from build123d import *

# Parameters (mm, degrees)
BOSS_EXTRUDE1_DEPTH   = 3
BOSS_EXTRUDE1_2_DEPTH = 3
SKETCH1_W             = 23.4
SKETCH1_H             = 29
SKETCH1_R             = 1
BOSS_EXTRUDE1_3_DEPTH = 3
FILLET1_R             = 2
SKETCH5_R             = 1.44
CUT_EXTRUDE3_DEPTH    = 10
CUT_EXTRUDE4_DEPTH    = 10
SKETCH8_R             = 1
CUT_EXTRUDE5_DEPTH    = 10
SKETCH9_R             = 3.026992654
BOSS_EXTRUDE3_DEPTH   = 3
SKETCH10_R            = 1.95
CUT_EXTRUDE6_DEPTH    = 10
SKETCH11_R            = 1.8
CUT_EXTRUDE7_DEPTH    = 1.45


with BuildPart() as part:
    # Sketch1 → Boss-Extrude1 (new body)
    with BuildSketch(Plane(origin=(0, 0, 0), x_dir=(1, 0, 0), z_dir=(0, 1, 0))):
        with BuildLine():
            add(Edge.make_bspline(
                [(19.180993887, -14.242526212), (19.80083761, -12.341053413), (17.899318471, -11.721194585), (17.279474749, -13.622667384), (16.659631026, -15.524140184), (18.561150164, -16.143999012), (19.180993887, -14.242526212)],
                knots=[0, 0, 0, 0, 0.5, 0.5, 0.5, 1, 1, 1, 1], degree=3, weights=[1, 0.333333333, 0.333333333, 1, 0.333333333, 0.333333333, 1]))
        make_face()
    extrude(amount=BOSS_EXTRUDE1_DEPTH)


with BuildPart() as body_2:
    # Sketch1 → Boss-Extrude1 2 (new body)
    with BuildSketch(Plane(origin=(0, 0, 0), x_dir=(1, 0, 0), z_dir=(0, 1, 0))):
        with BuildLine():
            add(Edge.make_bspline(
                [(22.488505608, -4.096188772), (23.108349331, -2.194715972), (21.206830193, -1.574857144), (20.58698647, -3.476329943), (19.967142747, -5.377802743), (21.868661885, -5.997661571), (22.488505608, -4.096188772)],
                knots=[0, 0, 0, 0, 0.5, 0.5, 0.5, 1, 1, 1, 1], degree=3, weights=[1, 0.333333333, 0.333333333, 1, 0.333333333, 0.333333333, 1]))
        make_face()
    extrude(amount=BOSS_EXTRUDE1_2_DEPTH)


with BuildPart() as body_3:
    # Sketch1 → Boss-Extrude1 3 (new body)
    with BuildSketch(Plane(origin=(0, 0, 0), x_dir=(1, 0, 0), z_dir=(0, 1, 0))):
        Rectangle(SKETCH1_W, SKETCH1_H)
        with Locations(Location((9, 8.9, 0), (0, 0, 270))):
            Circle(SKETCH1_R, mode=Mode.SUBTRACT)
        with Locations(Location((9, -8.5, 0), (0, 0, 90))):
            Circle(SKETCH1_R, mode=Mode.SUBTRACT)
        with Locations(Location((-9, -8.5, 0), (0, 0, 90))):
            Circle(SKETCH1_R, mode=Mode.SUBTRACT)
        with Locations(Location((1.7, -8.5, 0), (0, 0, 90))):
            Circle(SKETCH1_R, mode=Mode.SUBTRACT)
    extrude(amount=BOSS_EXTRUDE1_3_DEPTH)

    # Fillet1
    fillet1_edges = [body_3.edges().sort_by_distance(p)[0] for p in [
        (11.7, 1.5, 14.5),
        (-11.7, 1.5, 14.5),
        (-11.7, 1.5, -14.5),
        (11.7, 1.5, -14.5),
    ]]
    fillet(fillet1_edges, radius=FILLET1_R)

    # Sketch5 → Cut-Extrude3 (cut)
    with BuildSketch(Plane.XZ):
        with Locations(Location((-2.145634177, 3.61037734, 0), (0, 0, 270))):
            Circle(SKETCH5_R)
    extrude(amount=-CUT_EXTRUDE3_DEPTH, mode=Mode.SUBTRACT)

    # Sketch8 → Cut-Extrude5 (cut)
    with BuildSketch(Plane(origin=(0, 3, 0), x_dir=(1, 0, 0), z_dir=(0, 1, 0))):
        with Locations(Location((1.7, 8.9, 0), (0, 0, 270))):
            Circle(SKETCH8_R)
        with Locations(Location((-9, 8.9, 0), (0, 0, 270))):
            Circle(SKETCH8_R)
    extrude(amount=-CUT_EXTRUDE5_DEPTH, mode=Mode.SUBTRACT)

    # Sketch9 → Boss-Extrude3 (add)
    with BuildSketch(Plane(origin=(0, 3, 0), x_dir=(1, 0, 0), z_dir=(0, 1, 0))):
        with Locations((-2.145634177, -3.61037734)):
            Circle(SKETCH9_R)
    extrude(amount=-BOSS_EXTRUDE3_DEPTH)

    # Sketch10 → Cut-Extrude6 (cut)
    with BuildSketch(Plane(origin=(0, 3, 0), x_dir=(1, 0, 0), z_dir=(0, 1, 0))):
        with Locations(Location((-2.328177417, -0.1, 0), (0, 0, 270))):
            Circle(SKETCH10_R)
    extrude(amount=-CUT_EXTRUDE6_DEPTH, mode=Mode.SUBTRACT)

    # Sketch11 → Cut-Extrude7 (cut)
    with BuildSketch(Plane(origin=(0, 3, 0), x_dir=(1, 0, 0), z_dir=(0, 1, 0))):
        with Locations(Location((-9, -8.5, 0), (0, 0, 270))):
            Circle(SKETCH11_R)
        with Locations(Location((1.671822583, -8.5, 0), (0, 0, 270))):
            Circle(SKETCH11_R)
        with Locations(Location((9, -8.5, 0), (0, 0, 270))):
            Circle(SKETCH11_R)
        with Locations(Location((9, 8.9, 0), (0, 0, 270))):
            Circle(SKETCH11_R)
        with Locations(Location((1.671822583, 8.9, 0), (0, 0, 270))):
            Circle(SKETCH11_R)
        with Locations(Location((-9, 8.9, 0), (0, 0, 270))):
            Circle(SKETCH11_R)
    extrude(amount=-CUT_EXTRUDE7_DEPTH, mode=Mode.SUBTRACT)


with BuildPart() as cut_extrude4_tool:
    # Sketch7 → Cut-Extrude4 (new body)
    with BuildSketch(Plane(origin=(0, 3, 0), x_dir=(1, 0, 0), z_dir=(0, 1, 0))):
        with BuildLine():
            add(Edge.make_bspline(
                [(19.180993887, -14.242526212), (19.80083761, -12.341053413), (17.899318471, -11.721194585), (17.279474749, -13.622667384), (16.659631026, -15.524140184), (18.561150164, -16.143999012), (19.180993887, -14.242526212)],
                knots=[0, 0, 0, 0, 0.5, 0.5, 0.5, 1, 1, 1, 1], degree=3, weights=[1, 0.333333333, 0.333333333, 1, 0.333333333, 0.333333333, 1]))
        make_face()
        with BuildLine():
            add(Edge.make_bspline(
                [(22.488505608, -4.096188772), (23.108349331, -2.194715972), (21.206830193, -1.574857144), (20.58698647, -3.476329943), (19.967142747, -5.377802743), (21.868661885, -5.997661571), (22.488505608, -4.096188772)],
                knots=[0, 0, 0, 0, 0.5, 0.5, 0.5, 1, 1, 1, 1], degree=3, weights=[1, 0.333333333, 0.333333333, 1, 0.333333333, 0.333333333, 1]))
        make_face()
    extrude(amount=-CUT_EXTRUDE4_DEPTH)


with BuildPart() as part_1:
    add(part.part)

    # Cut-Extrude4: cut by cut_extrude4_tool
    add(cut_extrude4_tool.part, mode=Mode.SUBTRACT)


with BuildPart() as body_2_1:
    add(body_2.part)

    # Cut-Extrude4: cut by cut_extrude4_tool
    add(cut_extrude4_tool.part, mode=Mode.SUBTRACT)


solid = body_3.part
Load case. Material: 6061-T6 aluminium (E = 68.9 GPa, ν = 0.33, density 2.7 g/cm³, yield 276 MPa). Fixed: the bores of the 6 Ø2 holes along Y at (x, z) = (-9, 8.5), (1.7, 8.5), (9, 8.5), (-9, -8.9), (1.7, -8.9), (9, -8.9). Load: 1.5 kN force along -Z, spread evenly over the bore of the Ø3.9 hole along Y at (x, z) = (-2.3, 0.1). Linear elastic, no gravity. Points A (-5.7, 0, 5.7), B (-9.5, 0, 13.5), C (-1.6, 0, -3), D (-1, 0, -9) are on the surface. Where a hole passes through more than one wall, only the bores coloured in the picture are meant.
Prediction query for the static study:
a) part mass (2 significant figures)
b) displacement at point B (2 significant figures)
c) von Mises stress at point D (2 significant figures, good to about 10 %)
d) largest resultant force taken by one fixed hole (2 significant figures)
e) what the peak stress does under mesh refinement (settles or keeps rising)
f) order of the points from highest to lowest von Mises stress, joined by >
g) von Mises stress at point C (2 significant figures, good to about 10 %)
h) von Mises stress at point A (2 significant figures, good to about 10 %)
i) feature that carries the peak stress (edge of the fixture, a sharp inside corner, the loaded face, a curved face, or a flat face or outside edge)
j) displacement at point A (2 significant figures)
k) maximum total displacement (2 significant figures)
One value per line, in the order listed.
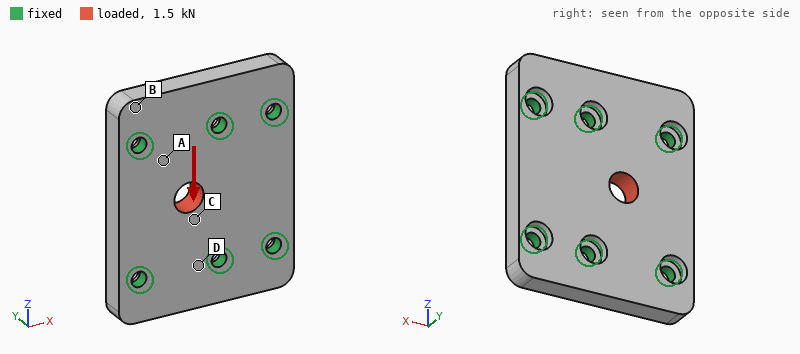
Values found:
5.1 g
1.7 µm
14 MPa
370 N
keeps rising
C > A > D > B
38 MPa
26 MPa
edge of the fixture
1.8 µm
4.4 µm
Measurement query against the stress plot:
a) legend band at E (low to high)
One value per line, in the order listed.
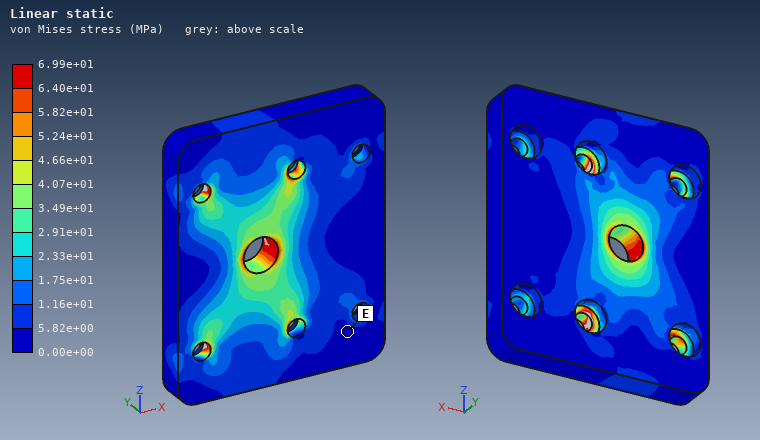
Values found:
0.00e+00 to 5.82e+00 MPa
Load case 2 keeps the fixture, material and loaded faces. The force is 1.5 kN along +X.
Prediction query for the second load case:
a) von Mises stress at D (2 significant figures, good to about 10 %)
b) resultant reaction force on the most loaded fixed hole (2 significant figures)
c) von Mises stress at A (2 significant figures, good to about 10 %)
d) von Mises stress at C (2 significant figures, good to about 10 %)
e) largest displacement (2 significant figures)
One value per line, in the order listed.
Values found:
16 MPa
330 N
30 MPa
34 MPa
6.0 µm
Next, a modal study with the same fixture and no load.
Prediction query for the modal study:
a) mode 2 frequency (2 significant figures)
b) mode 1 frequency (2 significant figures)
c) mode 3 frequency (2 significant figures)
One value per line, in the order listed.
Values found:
40 kHz
32 kHz
41 kHz
